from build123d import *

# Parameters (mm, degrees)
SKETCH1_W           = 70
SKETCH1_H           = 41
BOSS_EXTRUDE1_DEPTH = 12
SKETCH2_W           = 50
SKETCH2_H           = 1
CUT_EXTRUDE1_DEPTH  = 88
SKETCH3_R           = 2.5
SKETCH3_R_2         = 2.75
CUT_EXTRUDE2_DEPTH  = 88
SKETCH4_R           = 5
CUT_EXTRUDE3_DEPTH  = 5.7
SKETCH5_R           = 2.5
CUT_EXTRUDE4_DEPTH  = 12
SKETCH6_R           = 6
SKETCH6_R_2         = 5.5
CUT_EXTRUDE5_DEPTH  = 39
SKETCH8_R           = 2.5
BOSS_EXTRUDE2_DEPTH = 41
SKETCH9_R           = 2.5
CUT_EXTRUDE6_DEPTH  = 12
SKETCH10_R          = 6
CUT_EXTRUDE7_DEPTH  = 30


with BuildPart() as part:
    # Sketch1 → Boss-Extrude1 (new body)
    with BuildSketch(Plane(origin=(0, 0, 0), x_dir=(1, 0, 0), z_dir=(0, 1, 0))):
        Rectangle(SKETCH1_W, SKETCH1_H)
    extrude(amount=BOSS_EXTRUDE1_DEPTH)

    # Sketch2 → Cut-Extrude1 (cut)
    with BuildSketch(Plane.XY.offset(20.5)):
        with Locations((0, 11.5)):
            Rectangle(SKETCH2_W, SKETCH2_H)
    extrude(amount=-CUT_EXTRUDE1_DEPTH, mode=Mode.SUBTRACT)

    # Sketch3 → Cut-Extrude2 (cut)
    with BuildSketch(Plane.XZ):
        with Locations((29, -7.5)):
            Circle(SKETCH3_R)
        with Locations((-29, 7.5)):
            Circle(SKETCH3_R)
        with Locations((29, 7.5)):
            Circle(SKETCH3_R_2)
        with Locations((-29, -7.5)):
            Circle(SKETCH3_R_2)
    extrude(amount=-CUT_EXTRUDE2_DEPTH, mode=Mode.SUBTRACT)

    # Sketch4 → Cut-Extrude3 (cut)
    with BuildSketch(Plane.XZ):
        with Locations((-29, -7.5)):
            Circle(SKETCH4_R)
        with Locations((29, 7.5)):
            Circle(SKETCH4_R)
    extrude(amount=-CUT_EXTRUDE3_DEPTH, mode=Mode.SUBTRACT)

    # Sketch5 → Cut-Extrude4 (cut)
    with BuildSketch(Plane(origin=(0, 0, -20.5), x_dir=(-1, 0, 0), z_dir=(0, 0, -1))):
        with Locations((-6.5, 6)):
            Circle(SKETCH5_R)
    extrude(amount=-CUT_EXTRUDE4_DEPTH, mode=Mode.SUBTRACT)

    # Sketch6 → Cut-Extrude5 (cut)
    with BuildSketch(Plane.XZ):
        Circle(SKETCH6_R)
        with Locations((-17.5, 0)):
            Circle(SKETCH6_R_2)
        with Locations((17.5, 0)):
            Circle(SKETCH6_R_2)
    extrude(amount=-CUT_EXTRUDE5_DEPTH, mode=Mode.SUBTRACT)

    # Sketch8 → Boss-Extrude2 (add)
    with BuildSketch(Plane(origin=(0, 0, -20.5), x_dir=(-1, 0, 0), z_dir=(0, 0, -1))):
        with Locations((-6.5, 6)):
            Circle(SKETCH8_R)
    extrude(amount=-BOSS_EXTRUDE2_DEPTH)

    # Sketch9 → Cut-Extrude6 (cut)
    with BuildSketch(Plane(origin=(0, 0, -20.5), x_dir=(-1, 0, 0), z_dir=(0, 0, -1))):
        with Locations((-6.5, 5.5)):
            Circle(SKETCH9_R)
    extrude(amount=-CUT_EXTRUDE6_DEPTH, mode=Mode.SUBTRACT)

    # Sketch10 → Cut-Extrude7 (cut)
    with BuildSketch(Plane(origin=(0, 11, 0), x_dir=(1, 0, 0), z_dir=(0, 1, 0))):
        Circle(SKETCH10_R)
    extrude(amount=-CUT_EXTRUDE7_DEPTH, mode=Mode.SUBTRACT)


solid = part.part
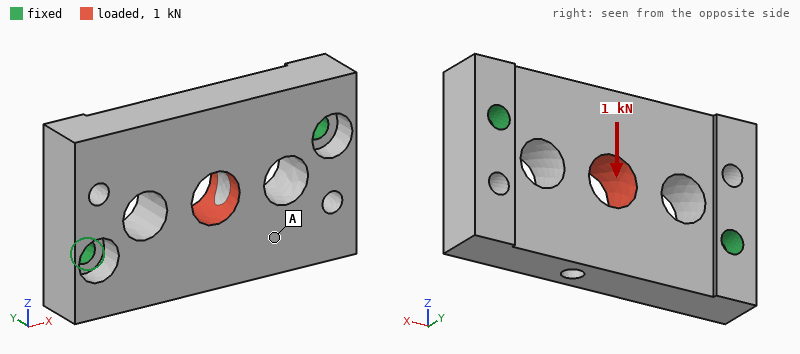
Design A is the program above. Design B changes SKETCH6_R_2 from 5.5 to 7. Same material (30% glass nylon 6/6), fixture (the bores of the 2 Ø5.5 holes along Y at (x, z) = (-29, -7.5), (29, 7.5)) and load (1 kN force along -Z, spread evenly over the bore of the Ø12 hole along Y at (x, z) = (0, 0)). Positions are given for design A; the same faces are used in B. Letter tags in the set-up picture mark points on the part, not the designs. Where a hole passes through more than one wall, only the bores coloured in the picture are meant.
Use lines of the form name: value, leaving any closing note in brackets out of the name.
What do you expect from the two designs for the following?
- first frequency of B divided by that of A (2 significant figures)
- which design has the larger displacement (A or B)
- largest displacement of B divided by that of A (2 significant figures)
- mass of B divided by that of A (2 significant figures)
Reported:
first frequency of B divided by that of A: 0.98
which design has the larger displacement: B
largest displacement of B divided by that of A: 1.1
mass of B divided by that of A: 0.95
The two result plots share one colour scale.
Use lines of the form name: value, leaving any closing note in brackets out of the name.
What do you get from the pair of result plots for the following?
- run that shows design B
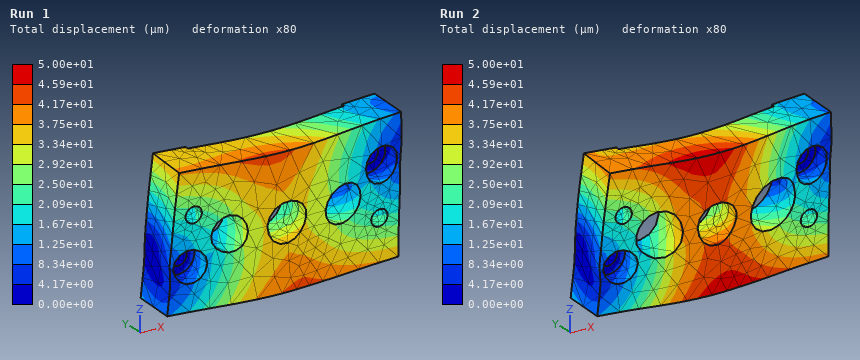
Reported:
run that shows design B: Run 2
